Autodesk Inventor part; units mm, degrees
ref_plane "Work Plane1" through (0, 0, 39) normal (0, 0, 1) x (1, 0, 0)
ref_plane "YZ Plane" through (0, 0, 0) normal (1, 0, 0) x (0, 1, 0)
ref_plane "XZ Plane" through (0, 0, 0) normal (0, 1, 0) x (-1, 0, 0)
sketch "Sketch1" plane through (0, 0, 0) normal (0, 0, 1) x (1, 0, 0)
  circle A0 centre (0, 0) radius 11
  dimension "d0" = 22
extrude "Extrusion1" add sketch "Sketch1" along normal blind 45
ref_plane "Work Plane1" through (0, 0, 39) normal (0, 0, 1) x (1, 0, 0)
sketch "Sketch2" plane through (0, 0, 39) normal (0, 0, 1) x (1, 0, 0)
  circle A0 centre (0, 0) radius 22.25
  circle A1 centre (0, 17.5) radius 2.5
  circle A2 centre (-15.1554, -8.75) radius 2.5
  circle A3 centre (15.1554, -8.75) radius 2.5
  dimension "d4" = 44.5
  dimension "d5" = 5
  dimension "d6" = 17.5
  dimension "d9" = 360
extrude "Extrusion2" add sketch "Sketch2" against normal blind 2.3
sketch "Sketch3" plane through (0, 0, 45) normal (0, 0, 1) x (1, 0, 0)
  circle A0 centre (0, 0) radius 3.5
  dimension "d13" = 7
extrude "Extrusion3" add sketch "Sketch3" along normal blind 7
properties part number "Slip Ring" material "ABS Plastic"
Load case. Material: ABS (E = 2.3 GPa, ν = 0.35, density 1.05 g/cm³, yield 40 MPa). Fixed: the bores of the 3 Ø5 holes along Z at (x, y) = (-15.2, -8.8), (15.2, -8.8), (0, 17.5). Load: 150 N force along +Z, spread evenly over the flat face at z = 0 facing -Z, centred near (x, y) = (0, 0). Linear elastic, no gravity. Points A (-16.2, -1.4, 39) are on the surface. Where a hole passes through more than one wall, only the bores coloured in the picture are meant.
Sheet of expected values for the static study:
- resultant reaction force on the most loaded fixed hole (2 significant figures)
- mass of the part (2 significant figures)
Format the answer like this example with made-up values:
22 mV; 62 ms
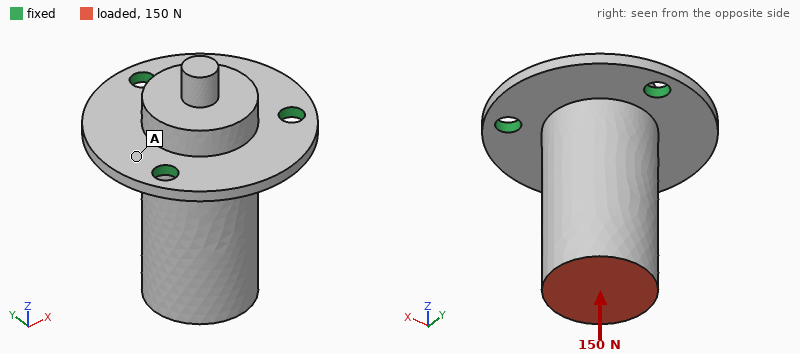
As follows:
50 N; 21 g
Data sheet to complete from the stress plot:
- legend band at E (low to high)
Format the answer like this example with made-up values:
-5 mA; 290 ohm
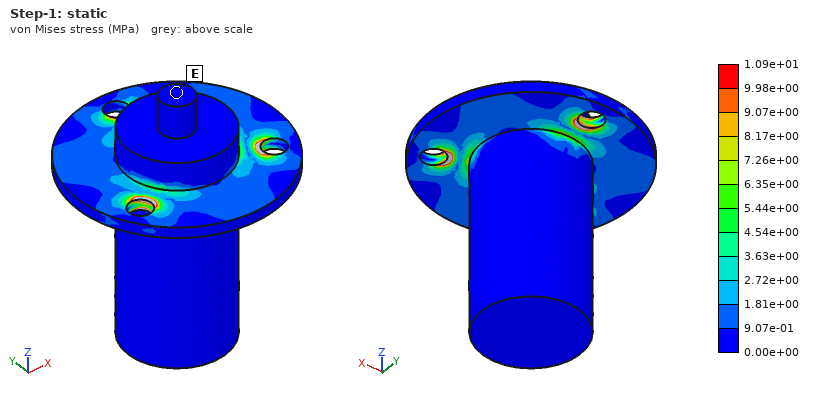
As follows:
0.00e+00 to 9.07e-01 MPa
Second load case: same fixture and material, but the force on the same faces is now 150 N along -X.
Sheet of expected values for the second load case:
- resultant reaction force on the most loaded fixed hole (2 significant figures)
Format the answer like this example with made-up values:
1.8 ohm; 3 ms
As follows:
230 N
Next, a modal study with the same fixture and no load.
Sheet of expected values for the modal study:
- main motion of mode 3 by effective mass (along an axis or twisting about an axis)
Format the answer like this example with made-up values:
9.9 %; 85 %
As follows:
along Z
